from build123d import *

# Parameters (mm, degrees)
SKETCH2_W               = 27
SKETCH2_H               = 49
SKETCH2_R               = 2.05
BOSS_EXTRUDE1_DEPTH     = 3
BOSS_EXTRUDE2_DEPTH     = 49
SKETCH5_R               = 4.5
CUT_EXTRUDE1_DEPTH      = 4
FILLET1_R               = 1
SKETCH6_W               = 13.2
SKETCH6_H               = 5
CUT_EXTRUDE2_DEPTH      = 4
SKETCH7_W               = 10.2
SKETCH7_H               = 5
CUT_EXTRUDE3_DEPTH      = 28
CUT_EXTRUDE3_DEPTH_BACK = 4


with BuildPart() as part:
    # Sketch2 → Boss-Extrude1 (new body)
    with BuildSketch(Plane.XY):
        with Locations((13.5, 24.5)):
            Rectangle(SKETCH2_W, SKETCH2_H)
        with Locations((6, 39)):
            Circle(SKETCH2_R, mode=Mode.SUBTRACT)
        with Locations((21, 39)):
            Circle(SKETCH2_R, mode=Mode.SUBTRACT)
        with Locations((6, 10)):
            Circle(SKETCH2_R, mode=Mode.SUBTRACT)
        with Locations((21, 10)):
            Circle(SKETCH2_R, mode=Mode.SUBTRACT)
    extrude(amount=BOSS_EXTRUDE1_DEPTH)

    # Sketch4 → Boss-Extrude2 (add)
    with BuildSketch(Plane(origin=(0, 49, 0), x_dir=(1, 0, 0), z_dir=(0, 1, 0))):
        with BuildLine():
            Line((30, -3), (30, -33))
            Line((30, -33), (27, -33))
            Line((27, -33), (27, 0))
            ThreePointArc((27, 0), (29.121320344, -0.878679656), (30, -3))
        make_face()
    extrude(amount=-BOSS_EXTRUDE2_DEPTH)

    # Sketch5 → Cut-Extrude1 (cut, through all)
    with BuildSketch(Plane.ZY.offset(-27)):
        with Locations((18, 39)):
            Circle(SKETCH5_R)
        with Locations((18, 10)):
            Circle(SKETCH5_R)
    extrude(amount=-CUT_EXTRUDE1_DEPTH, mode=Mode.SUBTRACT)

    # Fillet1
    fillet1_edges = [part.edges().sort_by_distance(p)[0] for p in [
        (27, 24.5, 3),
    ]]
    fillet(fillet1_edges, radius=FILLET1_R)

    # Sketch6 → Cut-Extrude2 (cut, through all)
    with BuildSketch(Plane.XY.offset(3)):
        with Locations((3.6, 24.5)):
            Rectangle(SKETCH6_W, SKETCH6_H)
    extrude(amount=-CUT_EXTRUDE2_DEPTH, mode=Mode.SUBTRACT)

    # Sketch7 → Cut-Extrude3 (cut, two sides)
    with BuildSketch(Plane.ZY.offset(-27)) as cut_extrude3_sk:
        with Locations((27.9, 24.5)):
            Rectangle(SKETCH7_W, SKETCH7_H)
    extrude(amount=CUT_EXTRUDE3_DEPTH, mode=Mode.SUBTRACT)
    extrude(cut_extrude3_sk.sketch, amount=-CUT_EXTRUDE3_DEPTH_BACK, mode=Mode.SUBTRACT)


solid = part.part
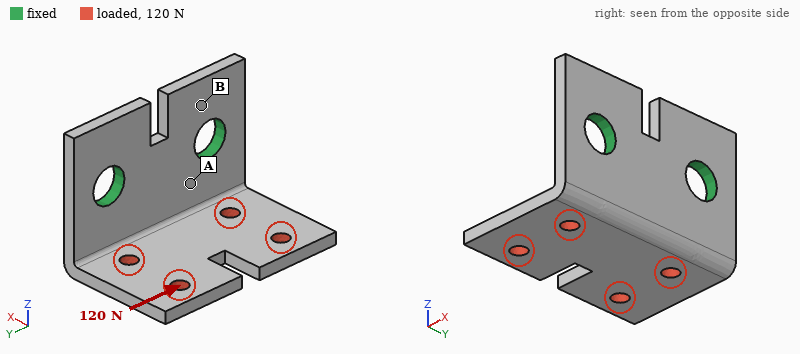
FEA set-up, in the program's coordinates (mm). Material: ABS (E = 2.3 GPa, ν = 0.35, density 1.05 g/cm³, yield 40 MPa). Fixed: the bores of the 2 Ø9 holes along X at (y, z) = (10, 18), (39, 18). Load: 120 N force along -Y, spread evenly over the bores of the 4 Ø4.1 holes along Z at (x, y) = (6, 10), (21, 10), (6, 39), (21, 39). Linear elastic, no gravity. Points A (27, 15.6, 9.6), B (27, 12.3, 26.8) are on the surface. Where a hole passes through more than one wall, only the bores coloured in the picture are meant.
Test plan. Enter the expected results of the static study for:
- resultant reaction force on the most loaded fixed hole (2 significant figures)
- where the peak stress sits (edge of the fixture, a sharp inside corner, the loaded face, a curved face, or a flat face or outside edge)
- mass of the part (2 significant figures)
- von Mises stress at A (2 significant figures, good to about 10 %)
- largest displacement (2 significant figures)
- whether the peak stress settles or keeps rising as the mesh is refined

94 N
edge of the fixture
8.3 g
7.5 MPa
0.68 mm
keeps rising
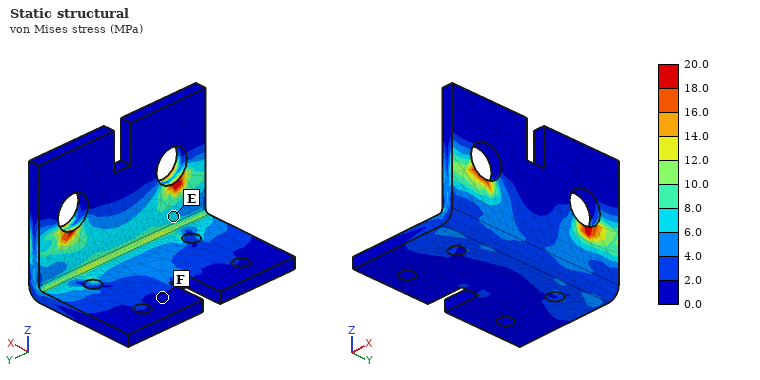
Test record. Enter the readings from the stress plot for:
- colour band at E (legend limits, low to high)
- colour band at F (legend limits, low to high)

6.0 to 8.0 MPa
0.0 to 2.0 MPa
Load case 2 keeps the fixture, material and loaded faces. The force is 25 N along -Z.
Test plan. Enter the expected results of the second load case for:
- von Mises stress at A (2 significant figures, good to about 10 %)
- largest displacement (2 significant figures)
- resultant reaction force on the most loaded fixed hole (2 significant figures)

4.7 MPa
0.78 mm
13 N
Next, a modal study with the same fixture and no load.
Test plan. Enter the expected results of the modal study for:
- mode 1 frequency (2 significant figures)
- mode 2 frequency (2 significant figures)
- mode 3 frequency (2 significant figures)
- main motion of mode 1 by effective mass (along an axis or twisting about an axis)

560 Hz
950 Hz
1500 Hz
along Z
